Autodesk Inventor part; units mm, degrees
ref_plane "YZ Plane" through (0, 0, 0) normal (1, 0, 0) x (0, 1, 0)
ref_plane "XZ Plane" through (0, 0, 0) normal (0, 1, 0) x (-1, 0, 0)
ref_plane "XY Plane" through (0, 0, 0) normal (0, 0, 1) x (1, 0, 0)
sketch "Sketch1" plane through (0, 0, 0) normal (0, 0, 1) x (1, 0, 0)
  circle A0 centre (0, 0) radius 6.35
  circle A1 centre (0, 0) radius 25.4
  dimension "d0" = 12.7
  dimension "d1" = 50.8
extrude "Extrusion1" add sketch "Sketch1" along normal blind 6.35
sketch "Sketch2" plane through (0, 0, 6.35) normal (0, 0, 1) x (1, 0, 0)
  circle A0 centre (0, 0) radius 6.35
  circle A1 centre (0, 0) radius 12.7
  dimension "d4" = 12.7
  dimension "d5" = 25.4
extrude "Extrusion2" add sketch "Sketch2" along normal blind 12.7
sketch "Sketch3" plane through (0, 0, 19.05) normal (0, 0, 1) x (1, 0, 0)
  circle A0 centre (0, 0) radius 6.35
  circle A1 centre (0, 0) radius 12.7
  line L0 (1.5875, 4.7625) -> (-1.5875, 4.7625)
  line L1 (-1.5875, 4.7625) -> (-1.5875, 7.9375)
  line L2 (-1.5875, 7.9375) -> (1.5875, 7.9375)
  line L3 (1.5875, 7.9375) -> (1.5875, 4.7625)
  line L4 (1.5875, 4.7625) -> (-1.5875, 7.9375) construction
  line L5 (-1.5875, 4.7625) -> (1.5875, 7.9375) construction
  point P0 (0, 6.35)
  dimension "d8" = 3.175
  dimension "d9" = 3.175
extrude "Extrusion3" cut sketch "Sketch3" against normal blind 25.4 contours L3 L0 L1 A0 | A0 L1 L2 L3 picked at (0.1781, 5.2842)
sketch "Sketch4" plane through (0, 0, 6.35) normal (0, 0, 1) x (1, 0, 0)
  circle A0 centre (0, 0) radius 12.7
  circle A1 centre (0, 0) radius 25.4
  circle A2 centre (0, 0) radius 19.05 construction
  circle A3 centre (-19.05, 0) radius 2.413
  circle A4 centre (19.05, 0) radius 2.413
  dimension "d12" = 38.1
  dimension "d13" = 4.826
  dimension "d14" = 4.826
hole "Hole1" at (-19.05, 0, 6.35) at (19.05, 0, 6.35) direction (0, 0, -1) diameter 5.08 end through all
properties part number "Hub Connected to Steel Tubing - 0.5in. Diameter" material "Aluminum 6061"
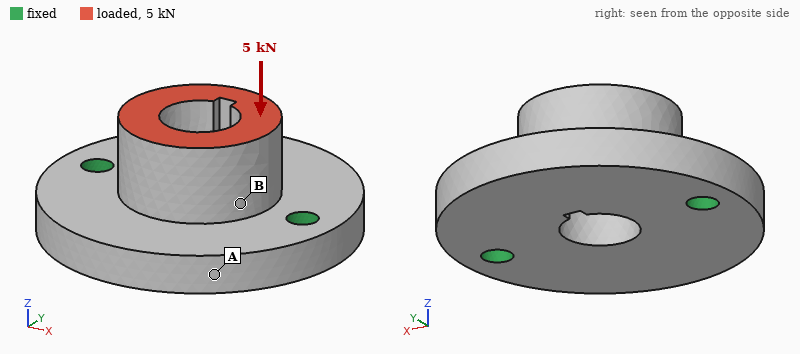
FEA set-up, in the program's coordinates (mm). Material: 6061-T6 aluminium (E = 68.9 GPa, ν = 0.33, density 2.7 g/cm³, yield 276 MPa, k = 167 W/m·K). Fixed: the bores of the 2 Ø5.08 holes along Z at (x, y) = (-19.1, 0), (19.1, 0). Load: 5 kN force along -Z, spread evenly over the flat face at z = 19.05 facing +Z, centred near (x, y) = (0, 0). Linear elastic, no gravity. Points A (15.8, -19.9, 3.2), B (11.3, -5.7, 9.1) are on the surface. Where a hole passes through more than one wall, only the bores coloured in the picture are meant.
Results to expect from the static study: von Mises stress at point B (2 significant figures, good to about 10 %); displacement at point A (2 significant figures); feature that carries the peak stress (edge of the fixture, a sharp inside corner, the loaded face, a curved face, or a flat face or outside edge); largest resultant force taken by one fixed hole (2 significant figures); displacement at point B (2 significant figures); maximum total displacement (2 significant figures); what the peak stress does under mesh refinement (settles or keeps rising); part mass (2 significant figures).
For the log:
40 MPa
16 µm
edge of the fixture
2.6 kN
16 µm
27 µm
keeps rising
45 g
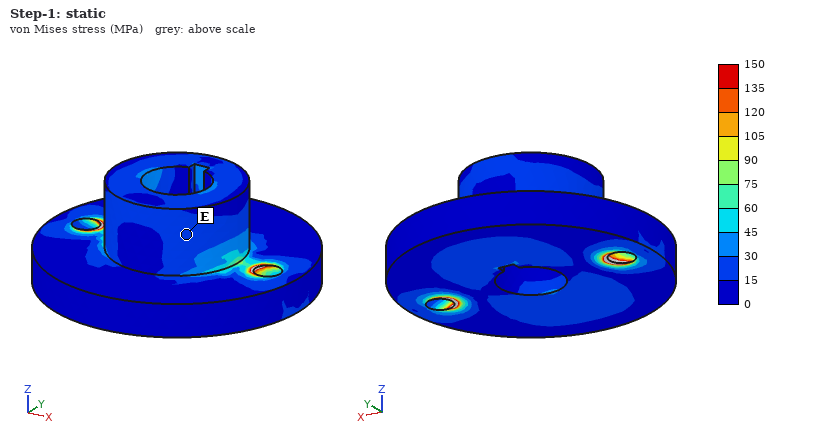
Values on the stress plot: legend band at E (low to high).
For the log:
15 to 30 MPa
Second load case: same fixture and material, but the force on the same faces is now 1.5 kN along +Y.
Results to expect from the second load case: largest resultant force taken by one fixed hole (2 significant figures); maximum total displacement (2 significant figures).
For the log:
750 N
49 µm
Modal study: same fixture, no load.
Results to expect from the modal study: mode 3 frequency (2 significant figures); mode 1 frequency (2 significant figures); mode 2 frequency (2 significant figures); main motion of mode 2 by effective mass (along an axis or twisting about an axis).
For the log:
20 kHz
6700 Hz
12 kHz
along Z
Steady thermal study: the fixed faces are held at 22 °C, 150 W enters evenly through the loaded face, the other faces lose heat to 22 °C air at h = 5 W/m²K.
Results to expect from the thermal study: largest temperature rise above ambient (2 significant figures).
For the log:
64 K
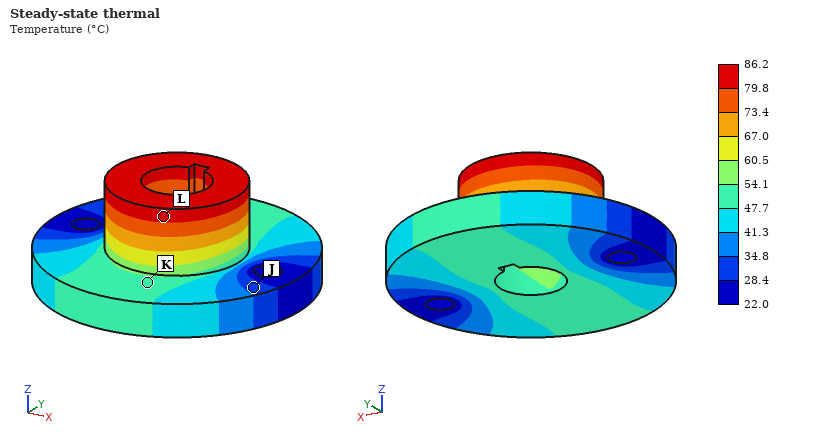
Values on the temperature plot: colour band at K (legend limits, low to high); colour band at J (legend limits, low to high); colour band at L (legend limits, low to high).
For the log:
47.7 to 54.1 °C
28.4 to 34.8 °C
79.8 to 86.2 °C
